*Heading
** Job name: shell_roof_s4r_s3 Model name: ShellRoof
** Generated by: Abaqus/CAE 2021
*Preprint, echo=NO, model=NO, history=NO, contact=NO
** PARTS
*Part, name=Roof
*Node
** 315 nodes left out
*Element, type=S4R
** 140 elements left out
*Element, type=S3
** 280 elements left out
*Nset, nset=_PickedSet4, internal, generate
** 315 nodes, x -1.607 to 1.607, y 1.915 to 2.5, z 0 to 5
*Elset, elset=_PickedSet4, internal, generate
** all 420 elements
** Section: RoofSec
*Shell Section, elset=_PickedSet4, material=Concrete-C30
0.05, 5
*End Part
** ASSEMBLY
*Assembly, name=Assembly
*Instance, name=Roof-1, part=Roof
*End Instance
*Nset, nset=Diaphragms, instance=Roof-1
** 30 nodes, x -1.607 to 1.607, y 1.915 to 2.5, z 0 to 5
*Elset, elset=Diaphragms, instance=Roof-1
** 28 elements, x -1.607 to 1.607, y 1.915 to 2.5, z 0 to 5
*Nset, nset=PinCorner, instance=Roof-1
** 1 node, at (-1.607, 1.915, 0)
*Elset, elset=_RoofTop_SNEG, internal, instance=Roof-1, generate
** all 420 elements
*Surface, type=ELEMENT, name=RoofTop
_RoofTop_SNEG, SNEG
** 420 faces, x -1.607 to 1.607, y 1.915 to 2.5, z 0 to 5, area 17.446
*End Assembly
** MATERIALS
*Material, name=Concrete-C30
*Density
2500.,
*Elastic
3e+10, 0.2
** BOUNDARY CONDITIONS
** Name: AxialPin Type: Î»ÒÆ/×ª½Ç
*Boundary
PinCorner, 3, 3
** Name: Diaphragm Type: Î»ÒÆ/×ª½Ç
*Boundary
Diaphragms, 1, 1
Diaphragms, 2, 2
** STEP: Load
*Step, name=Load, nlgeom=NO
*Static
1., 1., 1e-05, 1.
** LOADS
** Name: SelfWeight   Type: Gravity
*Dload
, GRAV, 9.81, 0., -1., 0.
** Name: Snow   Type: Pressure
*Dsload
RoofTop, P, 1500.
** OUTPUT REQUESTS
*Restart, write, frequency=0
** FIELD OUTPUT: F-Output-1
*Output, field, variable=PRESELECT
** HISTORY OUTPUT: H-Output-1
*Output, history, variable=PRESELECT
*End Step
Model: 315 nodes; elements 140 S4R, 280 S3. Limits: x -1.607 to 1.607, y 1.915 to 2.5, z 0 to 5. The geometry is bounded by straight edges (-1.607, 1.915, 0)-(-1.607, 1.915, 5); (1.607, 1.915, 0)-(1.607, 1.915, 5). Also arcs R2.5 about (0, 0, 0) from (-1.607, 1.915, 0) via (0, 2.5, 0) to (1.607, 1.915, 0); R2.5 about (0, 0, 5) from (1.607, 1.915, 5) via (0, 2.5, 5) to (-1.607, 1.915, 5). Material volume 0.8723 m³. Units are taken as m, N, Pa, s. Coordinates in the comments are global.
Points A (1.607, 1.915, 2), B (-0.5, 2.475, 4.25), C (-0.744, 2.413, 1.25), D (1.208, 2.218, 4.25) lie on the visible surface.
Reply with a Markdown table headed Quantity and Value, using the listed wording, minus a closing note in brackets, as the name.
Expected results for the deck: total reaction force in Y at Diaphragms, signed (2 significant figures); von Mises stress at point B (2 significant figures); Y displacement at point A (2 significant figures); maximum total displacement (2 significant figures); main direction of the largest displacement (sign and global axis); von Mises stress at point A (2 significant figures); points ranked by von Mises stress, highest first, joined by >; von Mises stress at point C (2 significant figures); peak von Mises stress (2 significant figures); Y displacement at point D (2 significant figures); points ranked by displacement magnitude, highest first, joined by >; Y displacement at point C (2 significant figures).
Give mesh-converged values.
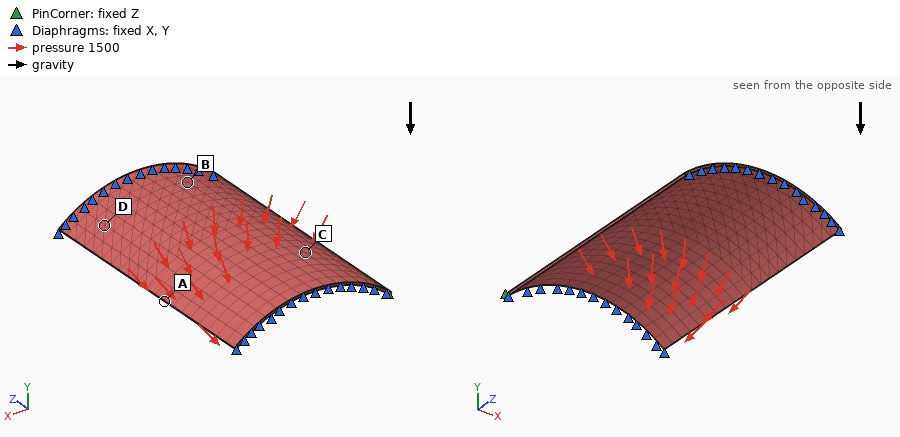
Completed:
| Quantity | Value |
|---|---|
| total reaction force in Y at Diaphragms, signed | 46000 N |
| von Mises stress at point B | 1.4e+06 Pa |
| Y displacement at point A | -0.0026 m |
| maximum total displacement | 0.0030 m |
| main direction of the largest displacement | -Y |
| von Mises stress at point A | 2.8e+06 Pa |
| points ranked by von Mises stress, highest first, joined by > | A > D > C > B |
| von Mises stress at point C | 1.7e+06 Pa |
| peak von Mises stress | 3.7e+06 Pa |
| Y displacement at point D | -8.6e-04 m |
| points ranked by displacement magnitude, highest first, joined by > | A > D > C > B |
| Y displacement at point C | -5.5e-04 m |
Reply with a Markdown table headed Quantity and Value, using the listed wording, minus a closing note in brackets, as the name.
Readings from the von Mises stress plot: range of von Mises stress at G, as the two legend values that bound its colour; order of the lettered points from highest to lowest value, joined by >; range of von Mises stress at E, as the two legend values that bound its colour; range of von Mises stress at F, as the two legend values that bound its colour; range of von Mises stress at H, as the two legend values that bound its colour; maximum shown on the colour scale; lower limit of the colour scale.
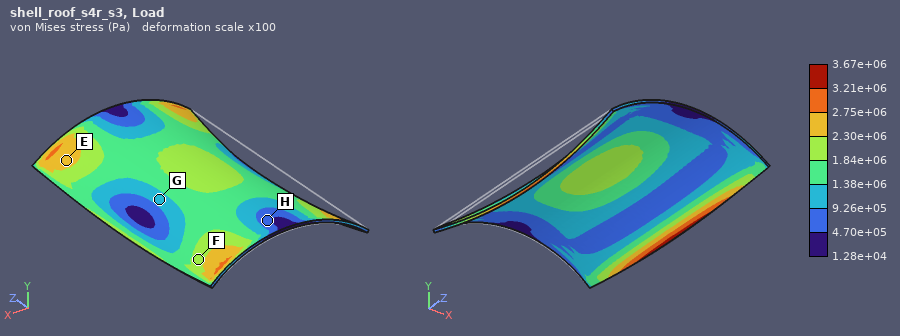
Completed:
| Quantity | Value |
|---|---|
| range of von Mises stress at G, as the two legend values that bound its colour | 9.26e+05 to 1.38e+06 Pa |
| order of the lettered points from highest to lowest value, joined by > | E > F > G > H |
| range of von Mises stress at E, as the two legend values that bound its colour | 2.30e+06 to 2.75e+06 Pa |
| range of von Mises stress at F, as the two legend values that bound its colour | 1.84e+06 to 2.30e+06 Pa |
| range of von Mises stress at H, as the two legend values that bound its colour | 4.70e+05 to 9.26e+05 Pa |
| maximum shown on the colour scale | 3.67e+06 Pa |
| lower limit of the colour scale | 1.28e+04 Pa |
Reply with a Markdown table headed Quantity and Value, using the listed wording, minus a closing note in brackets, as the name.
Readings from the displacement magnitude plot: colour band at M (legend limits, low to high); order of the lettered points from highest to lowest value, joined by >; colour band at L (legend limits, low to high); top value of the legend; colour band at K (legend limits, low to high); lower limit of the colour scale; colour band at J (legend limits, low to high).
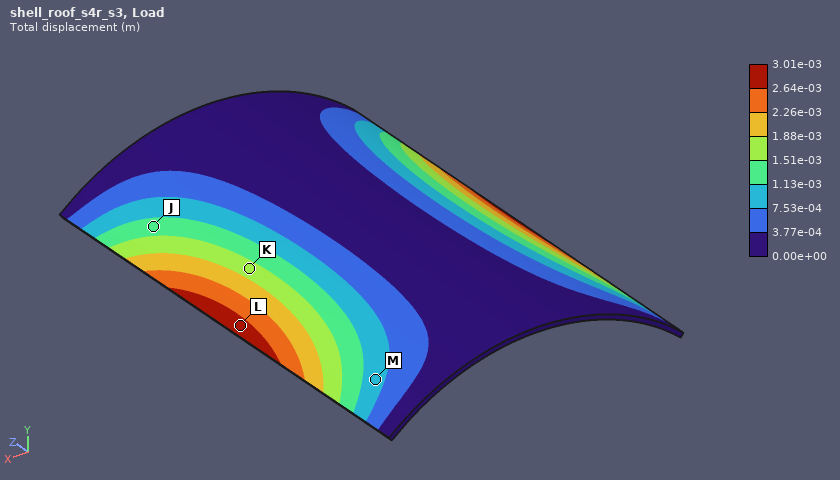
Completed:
| Quantity | Value |
|---|---|
| colour band at M | 7.53e-04 to 1.13e-03 m |
| order of the lettered points from highest to lowest value, joined by > | L > K > J > M |
| colour band at L | 2.64e-03 to 3.01e-03 m |
| top value of the legend | 3.01e-03 m |
| colour band at K | 1.51e-03 to 1.88e-03 m |
| lower limit of the colour scale | 0.00e+00 m |
| colour band at J | 1.13e-03 to 1.51e-03 m |
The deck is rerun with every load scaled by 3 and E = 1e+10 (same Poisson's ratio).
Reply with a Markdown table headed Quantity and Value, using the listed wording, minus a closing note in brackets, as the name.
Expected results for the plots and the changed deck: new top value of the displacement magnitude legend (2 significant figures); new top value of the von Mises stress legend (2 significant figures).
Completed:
| Quantity | Value |
|---|---|
| new top value of the displacement magnitude legend | 0.027 m |
| new top value of the von Mises stress legend | 1.1e+07 Pa |
